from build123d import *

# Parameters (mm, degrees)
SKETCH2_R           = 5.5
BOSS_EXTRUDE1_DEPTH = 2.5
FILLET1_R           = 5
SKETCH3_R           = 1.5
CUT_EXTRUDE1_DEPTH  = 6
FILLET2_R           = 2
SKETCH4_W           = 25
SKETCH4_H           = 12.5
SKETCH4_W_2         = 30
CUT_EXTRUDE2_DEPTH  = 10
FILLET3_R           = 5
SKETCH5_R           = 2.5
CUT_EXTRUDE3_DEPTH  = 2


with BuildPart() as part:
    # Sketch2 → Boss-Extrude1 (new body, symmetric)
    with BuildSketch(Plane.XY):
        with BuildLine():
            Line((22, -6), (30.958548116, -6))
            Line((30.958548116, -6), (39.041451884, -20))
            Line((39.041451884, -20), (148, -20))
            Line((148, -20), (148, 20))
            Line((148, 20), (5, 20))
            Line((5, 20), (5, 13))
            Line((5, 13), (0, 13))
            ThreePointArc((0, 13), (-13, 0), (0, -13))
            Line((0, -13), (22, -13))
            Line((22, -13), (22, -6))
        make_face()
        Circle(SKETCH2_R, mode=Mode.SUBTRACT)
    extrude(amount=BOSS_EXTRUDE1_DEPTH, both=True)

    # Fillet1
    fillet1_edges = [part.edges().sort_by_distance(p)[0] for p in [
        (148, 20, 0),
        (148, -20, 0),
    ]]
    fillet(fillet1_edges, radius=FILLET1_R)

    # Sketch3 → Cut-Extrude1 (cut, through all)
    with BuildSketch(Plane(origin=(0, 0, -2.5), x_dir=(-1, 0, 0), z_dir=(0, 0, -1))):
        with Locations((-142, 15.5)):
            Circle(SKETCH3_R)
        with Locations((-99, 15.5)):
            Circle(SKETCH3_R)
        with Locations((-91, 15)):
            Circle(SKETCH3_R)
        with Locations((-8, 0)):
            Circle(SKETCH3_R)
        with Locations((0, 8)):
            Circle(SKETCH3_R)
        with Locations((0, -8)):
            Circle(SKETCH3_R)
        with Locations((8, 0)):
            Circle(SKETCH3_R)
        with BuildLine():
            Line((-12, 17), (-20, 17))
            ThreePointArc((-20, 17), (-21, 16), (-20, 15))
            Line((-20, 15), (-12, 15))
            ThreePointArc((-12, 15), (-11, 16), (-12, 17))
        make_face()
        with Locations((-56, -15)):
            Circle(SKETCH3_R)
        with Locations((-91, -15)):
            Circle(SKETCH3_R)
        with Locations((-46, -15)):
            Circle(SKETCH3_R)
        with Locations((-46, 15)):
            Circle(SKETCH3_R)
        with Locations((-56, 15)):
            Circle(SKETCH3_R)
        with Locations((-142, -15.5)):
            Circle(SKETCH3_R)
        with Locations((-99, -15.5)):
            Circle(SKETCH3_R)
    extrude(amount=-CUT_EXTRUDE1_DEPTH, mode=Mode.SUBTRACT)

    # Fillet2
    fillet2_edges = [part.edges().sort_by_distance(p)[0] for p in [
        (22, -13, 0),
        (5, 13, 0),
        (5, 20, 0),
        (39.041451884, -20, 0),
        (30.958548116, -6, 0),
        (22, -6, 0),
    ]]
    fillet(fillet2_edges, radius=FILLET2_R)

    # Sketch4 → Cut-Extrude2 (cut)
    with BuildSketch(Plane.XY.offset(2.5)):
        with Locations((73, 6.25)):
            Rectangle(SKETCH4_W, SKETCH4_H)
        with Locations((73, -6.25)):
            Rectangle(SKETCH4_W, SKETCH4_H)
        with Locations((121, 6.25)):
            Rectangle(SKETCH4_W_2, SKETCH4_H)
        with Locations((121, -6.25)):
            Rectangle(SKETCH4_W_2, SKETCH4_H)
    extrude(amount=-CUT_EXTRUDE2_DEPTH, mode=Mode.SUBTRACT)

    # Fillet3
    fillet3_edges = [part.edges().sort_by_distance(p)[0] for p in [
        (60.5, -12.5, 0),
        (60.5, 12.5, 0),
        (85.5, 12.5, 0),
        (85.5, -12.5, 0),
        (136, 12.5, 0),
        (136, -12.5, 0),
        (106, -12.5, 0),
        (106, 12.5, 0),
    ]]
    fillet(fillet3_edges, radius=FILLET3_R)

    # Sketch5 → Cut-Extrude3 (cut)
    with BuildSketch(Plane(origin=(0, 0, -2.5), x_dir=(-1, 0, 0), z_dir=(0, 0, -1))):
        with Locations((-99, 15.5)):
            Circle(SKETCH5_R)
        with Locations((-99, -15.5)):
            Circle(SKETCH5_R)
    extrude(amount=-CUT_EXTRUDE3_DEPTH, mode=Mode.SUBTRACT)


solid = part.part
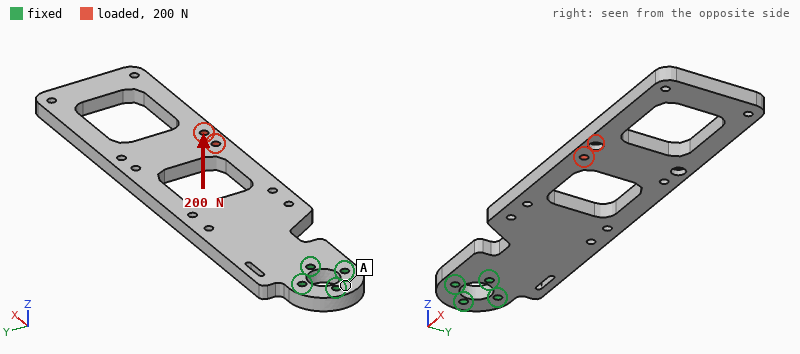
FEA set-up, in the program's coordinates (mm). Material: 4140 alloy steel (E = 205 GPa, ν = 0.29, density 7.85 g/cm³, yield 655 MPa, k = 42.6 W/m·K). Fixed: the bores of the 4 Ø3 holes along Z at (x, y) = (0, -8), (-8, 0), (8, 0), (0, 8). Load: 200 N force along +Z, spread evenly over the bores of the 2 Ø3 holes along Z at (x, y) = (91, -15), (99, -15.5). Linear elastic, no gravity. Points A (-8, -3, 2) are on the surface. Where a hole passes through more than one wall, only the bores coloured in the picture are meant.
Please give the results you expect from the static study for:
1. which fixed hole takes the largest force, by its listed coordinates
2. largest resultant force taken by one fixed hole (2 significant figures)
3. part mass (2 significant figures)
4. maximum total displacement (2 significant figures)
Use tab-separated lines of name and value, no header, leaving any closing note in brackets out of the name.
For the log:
which fixed hole takes the largest force, by its listed coordinates	(8, 0)
largest resultant force taken by one fixed hole	1.2 kN
part mass	170 g
maximum total displacement	1.6 mm
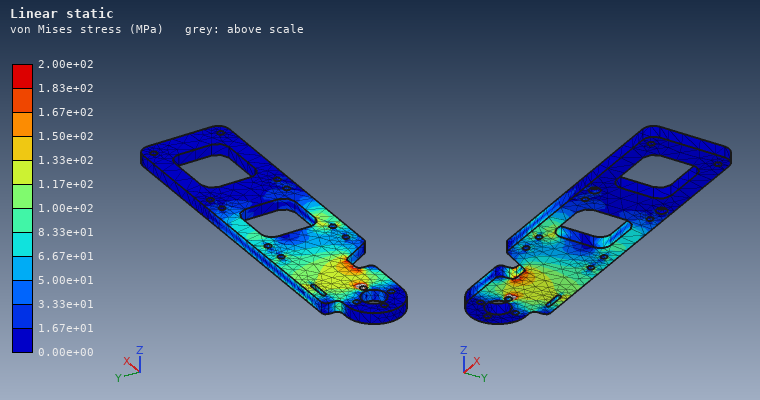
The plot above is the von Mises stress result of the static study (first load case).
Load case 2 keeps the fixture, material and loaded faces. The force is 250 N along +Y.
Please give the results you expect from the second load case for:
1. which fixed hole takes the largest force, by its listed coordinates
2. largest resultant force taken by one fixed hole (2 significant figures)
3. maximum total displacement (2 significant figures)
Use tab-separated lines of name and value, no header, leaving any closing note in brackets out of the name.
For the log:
which fixed hole takes the largest force, by its listed coordinates	(0, 8)
largest resultant force taken by one fixed hole	1.1 kN
maximum total displacement	83 µm
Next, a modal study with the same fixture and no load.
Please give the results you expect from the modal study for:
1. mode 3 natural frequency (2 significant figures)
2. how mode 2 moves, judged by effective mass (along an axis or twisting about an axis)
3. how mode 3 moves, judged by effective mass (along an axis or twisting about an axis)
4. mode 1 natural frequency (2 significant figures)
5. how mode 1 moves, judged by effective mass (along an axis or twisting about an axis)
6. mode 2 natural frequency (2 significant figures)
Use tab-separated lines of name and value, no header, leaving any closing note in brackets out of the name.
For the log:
mode 3 natural frequency	1100 Hz
how mode 2 moves, judged by effective mass	along Y
how mode 3 moves, judged by effective mass	along Z
mode 1 natural frequency	200 Hz
how mode 1 moves, judged by effective mass	along Z
mode 2 natural frequency	990 Hz
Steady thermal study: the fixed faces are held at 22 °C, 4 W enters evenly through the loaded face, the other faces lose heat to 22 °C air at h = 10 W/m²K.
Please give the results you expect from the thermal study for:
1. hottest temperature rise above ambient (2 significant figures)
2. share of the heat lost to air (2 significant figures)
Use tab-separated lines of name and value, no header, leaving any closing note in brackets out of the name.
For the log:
hottest temperature rise above ambient	44 K
share of the heat lost to air	60 %
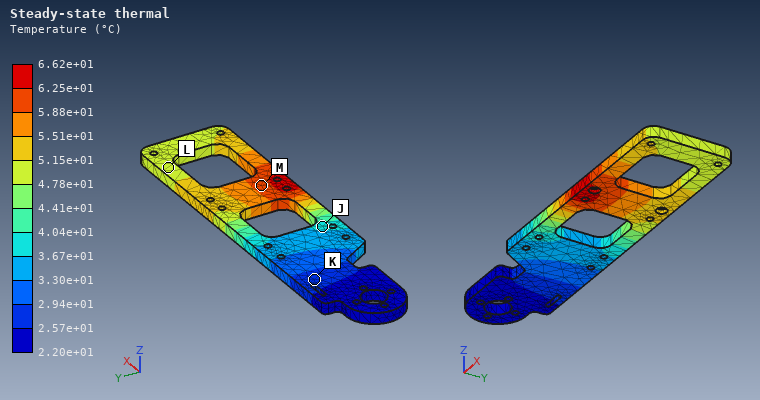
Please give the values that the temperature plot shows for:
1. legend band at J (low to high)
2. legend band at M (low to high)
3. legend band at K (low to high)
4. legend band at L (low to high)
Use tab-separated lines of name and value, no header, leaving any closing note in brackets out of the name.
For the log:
legend band at J	3.67e+01 to 4.04e+01 °C
legend band at M	5.88e+01 to 6.25e+01 °C
legend band at K	2.57e+01 to 2.94e+01 °C
legend band at L	4.78e+01 to 5.15e+01 °C
